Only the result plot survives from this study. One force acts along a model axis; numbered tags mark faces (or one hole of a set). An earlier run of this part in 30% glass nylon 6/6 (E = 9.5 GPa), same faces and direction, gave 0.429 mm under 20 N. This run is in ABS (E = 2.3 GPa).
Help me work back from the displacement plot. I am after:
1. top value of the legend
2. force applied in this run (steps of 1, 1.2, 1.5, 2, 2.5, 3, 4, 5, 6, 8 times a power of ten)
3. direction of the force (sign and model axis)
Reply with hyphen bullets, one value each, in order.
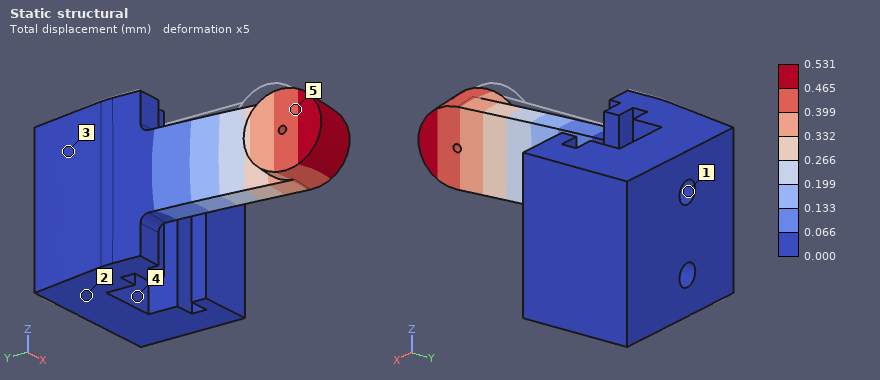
- 0.531 mm
- 6 N
- +X
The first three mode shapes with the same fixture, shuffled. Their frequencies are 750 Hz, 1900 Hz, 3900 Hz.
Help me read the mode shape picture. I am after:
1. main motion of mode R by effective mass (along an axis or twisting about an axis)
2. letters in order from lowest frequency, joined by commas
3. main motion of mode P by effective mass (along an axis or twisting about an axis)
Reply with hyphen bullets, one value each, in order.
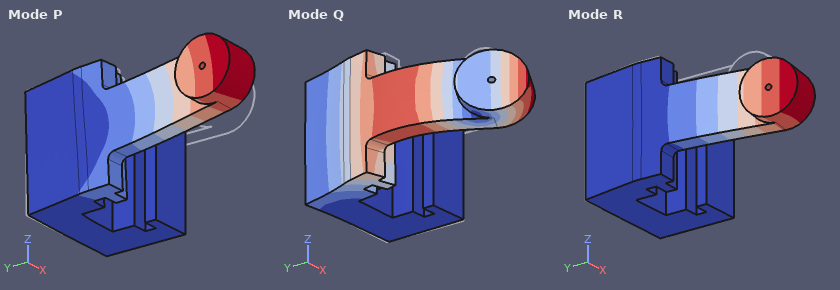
- along X
- R, P, Q
- along Z
